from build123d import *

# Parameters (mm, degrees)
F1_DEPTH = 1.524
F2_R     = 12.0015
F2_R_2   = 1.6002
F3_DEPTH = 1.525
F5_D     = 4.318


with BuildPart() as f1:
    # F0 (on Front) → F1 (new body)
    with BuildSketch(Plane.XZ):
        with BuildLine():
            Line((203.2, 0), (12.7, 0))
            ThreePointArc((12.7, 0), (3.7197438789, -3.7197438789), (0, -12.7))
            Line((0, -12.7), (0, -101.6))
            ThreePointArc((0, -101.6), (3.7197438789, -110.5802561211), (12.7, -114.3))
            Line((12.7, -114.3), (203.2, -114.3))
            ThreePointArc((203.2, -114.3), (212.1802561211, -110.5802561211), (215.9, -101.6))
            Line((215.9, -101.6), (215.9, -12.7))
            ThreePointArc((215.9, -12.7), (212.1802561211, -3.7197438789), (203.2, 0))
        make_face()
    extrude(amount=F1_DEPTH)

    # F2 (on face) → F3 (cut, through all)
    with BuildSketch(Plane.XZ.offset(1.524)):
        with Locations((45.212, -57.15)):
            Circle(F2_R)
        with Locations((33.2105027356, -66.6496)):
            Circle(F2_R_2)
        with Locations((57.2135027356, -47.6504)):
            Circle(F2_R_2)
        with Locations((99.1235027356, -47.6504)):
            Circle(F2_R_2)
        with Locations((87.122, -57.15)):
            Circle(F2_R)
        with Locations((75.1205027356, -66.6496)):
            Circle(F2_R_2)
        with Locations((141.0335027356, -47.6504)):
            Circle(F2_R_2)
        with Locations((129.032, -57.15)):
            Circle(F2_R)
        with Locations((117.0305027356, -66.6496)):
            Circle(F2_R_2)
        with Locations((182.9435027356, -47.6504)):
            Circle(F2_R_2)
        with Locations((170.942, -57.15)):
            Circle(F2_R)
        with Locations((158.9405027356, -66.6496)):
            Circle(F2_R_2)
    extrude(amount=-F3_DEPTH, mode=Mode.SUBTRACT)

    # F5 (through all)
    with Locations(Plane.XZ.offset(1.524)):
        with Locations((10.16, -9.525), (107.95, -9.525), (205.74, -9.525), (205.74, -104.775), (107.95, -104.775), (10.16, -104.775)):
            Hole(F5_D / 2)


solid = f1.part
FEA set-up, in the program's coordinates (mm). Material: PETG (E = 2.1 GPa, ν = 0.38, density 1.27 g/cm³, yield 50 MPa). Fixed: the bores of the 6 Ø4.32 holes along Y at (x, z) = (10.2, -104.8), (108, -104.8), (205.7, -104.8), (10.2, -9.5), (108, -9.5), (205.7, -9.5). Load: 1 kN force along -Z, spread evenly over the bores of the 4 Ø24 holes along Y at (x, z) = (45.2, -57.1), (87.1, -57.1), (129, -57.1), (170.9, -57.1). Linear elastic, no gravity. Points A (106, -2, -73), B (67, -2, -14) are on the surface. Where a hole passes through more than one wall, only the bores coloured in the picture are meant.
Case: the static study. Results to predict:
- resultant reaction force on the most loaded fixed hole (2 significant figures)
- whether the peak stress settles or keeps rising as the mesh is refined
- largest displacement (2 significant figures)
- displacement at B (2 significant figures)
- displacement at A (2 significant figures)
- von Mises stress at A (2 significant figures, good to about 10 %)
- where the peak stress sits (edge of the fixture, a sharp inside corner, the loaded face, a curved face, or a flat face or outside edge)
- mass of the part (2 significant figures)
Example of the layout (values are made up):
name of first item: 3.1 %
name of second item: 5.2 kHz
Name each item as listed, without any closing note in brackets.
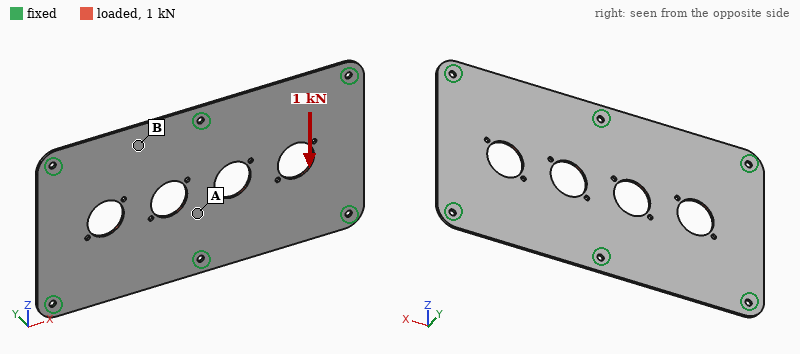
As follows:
resultant reaction force on the most loaded fixed hole: 270 N
whether the peak stress settles or keeps rising as the mesh is refined: keeps rising
largest displacement: 0.14 mm
displacement at B: 0.11 mm
displacement at A: 0.086 mm
von Mises stress at A: 2.6 MPa
where the peak stress sits: edge of the fixture
mass of the part: 44 g
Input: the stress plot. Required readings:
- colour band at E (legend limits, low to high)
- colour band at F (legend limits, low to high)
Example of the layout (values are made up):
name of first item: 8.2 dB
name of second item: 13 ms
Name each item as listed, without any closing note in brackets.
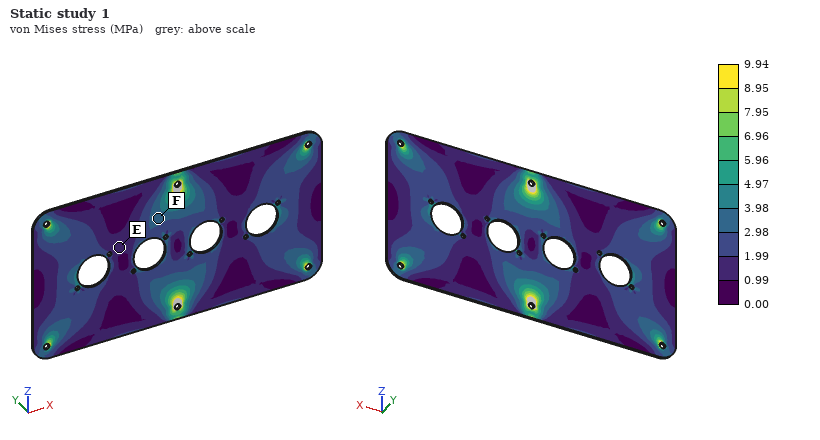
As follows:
colour band at E: 0.99 to 1.99 MPa
colour band at F: 2.98 to 3.98 MPa
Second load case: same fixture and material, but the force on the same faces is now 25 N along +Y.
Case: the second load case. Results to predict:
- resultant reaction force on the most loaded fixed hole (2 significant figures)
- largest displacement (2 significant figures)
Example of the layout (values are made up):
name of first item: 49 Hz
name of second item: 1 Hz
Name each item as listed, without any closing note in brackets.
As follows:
resultant reaction force on the most loaded fixed hole: 7.8 N
largest displacement: 2.5 mm
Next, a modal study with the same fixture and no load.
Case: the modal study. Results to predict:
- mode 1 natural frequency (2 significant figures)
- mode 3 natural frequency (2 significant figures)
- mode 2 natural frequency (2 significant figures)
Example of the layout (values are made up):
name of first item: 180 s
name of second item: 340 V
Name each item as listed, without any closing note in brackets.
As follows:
mode 1 natural frequency: 150 Hz
mode 3 natural frequency: 230 Hz
mode 2 natural frequency: 150 Hz
